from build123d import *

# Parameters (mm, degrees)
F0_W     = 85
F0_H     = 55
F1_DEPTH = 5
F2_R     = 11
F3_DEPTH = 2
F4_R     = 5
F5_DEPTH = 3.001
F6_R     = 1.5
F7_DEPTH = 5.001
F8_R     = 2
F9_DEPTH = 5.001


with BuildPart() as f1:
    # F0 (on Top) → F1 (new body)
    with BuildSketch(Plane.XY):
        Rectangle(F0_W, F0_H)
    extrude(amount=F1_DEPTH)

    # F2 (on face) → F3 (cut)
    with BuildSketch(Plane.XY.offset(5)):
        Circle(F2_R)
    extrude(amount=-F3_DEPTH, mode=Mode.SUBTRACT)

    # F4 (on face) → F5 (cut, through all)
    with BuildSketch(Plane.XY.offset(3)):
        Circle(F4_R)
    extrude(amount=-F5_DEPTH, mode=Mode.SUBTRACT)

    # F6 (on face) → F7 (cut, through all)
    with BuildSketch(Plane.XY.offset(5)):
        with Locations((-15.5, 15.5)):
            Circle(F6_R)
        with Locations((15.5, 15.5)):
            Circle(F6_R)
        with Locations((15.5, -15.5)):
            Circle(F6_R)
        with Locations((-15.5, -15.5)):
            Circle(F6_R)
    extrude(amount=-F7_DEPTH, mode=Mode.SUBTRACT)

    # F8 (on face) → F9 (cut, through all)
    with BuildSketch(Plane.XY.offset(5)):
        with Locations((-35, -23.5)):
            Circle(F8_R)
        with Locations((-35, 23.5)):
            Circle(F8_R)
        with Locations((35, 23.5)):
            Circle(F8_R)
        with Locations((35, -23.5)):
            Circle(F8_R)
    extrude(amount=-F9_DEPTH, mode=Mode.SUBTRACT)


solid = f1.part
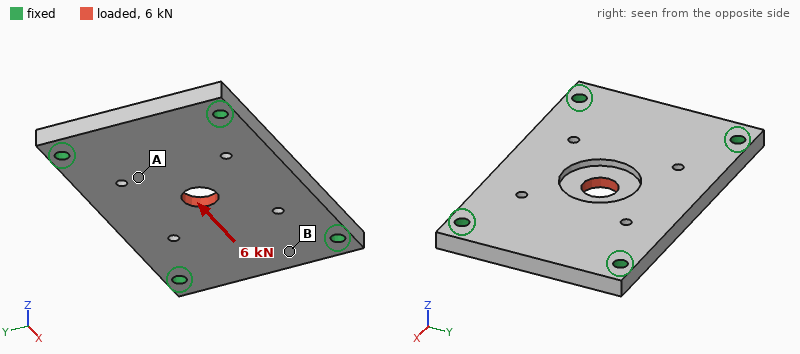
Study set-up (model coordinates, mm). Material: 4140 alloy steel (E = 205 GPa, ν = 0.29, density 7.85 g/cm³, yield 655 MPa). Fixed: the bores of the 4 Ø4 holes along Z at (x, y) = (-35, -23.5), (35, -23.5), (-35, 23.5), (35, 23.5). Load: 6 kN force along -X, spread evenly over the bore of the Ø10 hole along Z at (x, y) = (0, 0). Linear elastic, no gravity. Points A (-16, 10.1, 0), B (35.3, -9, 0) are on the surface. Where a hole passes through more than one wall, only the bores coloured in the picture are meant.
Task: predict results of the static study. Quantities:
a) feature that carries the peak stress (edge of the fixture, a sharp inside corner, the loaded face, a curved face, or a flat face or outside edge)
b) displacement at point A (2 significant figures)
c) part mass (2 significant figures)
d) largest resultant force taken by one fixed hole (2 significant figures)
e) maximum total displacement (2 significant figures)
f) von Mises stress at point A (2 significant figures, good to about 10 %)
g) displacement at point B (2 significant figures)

the loaded face
2.8 µm
170 g
1.6 kN
5.9 µm
27 MPa
2.1 µm
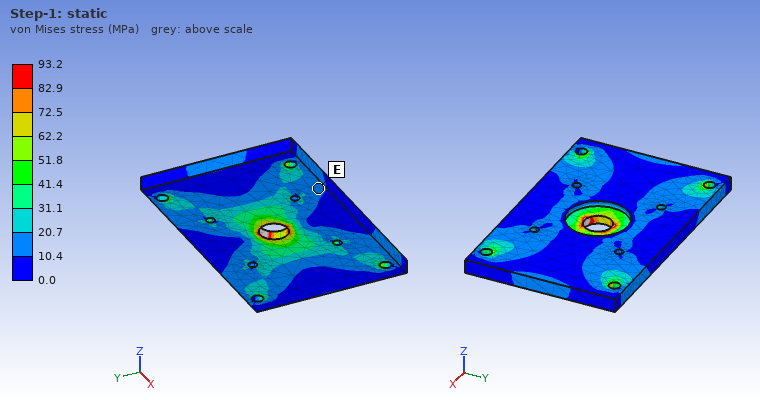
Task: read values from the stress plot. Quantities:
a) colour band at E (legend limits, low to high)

10.4 to 20.7 MPa
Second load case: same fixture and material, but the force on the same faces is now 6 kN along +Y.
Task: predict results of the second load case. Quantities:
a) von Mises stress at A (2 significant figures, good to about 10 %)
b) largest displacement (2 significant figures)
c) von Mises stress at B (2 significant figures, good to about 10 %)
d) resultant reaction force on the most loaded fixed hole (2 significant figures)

34 MPa
8.8 µm
12 MPa
1.9 kN
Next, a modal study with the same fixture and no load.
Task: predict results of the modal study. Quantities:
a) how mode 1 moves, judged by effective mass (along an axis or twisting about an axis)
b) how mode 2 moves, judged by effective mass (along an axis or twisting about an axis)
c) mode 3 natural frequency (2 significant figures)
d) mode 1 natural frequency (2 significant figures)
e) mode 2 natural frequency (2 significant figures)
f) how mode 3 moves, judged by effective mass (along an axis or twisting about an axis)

along Z
twisting about X
9700 Hz
4300 Hz
6700 Hz
twisting about Y
